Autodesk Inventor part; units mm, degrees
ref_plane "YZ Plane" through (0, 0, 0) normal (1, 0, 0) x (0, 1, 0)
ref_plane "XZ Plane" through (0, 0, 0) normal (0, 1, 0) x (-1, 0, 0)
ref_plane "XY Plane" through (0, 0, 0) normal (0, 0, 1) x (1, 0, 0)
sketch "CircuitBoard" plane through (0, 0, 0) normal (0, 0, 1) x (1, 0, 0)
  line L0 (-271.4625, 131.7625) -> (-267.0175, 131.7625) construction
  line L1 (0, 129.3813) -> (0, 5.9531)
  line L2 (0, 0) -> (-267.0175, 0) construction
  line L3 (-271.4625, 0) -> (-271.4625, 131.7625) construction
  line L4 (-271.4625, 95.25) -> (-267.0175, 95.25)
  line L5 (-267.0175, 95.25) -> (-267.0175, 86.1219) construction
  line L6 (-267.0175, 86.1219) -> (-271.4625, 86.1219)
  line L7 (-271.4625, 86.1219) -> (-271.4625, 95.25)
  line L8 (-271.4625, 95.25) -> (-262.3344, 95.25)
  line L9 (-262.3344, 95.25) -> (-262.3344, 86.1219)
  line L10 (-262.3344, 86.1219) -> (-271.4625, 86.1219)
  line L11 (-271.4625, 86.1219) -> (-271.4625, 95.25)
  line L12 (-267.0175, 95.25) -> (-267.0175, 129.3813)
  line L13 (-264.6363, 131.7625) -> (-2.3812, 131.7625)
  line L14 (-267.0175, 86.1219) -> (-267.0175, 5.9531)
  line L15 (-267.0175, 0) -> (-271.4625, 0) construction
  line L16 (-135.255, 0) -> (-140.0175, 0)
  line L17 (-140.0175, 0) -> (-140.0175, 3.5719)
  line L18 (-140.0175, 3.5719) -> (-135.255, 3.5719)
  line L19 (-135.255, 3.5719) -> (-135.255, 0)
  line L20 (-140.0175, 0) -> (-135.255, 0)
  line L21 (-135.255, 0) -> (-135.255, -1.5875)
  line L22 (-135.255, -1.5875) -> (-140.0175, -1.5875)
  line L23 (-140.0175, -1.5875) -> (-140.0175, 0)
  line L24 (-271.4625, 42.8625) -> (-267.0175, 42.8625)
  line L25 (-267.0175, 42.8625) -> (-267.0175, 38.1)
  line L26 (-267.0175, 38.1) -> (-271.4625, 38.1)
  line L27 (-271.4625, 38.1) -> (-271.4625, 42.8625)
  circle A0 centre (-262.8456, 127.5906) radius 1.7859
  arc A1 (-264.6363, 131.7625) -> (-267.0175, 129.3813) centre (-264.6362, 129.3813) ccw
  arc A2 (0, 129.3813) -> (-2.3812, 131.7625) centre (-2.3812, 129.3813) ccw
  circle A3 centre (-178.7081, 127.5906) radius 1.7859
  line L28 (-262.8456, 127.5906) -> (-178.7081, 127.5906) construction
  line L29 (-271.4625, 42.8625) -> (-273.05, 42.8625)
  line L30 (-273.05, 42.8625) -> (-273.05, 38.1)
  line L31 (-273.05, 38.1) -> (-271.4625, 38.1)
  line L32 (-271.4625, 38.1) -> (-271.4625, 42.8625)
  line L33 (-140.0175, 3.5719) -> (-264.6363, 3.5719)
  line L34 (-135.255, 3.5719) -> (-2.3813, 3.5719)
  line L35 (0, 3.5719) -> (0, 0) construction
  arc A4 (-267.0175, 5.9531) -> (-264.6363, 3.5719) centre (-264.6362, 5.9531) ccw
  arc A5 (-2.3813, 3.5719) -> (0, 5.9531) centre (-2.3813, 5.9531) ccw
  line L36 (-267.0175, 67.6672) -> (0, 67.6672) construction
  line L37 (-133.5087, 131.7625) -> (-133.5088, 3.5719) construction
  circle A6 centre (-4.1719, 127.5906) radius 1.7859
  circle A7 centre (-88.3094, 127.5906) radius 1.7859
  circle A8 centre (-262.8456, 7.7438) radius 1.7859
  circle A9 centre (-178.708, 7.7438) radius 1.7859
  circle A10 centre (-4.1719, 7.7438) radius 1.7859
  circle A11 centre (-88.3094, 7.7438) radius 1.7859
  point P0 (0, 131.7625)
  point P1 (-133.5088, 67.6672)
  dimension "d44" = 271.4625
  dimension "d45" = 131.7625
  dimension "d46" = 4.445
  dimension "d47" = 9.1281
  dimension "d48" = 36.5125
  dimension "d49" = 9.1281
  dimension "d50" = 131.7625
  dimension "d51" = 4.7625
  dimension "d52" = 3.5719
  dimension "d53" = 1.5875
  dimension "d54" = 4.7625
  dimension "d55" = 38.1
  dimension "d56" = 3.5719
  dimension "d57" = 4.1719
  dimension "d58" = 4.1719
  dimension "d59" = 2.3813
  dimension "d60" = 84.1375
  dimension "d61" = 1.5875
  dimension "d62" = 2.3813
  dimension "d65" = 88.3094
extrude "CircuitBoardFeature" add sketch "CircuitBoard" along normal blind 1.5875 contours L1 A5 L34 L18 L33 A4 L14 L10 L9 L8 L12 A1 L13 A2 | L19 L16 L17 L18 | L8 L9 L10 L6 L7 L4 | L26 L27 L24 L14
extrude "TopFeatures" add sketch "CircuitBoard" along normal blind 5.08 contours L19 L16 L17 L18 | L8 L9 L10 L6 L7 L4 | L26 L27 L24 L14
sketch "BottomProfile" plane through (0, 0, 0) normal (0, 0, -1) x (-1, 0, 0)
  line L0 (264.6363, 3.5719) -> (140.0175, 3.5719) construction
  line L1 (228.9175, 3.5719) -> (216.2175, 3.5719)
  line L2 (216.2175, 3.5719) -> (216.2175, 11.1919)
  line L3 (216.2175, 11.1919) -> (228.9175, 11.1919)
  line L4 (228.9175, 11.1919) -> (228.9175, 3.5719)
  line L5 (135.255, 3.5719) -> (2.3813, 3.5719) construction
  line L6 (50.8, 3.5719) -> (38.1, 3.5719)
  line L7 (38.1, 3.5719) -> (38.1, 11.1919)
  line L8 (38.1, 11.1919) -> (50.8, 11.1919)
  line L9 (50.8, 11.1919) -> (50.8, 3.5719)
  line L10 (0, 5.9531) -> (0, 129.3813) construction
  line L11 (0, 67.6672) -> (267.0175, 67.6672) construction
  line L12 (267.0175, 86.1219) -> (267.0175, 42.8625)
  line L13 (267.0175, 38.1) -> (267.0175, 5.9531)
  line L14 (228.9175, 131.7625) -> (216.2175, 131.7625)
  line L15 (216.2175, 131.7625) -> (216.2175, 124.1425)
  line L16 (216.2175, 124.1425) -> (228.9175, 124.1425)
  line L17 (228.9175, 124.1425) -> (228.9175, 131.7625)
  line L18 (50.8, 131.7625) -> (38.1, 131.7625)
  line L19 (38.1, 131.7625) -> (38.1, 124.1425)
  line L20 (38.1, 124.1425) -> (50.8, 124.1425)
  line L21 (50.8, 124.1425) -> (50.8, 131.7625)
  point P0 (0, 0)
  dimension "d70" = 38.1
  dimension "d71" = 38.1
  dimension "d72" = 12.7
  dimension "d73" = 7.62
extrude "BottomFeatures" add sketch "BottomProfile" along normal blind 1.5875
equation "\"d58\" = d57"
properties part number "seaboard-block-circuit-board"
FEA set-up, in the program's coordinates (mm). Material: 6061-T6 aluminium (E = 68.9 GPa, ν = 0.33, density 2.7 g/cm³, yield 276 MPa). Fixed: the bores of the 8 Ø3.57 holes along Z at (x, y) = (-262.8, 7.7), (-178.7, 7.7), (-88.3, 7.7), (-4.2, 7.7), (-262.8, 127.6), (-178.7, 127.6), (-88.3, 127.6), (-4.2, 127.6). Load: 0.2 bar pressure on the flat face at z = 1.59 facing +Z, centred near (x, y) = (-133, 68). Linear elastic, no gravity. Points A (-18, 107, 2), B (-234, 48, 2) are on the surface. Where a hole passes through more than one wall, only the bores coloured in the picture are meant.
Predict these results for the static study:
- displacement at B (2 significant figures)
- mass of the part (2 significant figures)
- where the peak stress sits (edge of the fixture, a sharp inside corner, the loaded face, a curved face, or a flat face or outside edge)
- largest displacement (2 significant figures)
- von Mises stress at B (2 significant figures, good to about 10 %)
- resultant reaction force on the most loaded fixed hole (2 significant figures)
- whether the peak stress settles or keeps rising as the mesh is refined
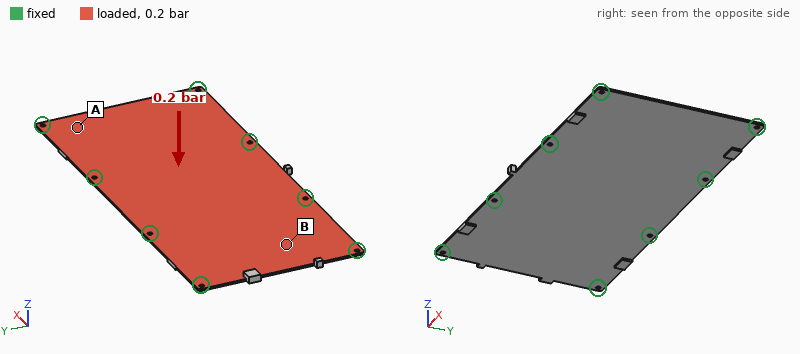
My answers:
0.69 mm
150 g
edge of the fixture
0.86 mm
27 MPa
120 N
keeps rising
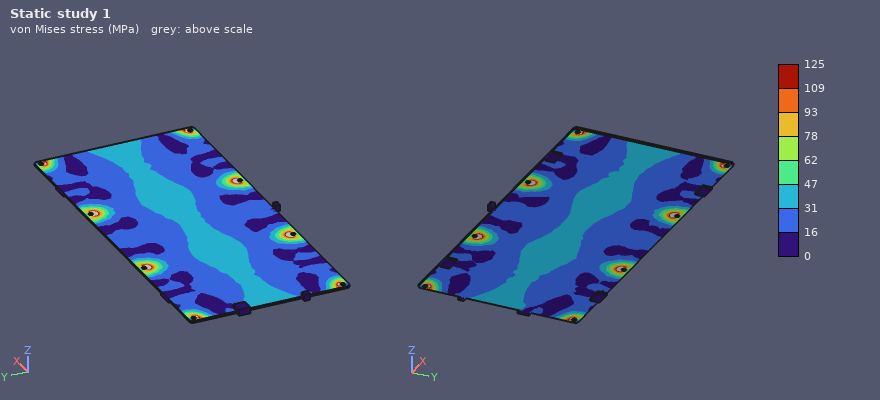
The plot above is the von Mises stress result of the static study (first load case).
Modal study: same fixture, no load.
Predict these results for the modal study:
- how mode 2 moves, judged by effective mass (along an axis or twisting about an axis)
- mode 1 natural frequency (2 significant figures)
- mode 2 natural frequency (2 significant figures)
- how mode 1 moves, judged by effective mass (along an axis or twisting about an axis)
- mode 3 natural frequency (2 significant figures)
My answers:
twisting about Y
430 Hz
470 Hz
along Z
550 Hz
